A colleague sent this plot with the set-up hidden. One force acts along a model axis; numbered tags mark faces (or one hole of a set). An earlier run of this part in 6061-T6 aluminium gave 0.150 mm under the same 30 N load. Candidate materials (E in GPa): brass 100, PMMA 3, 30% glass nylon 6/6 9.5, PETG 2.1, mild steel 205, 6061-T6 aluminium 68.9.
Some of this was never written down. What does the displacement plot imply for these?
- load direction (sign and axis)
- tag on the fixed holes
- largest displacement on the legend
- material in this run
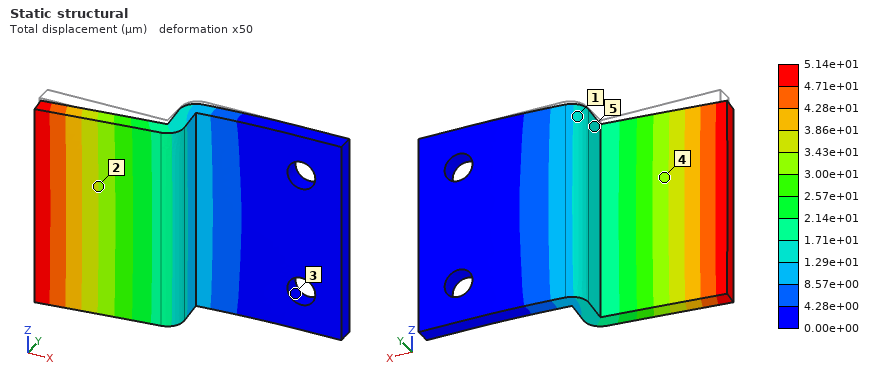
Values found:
-Y
3
5.14e+01 µm
mild steel
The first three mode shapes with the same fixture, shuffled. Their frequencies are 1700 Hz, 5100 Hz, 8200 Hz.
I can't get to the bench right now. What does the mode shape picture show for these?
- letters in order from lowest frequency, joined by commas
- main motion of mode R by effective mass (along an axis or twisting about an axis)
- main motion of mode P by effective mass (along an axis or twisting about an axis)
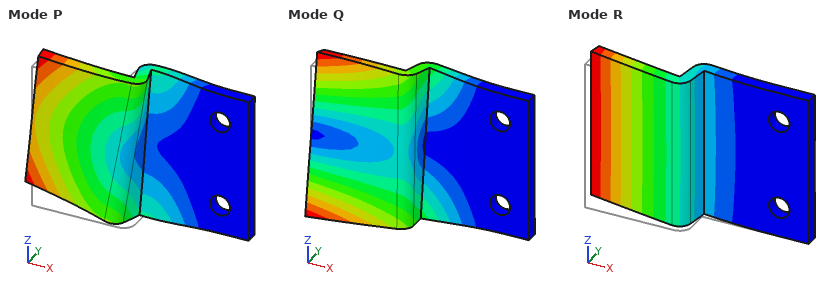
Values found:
R, Q, P
along Y
along Z
